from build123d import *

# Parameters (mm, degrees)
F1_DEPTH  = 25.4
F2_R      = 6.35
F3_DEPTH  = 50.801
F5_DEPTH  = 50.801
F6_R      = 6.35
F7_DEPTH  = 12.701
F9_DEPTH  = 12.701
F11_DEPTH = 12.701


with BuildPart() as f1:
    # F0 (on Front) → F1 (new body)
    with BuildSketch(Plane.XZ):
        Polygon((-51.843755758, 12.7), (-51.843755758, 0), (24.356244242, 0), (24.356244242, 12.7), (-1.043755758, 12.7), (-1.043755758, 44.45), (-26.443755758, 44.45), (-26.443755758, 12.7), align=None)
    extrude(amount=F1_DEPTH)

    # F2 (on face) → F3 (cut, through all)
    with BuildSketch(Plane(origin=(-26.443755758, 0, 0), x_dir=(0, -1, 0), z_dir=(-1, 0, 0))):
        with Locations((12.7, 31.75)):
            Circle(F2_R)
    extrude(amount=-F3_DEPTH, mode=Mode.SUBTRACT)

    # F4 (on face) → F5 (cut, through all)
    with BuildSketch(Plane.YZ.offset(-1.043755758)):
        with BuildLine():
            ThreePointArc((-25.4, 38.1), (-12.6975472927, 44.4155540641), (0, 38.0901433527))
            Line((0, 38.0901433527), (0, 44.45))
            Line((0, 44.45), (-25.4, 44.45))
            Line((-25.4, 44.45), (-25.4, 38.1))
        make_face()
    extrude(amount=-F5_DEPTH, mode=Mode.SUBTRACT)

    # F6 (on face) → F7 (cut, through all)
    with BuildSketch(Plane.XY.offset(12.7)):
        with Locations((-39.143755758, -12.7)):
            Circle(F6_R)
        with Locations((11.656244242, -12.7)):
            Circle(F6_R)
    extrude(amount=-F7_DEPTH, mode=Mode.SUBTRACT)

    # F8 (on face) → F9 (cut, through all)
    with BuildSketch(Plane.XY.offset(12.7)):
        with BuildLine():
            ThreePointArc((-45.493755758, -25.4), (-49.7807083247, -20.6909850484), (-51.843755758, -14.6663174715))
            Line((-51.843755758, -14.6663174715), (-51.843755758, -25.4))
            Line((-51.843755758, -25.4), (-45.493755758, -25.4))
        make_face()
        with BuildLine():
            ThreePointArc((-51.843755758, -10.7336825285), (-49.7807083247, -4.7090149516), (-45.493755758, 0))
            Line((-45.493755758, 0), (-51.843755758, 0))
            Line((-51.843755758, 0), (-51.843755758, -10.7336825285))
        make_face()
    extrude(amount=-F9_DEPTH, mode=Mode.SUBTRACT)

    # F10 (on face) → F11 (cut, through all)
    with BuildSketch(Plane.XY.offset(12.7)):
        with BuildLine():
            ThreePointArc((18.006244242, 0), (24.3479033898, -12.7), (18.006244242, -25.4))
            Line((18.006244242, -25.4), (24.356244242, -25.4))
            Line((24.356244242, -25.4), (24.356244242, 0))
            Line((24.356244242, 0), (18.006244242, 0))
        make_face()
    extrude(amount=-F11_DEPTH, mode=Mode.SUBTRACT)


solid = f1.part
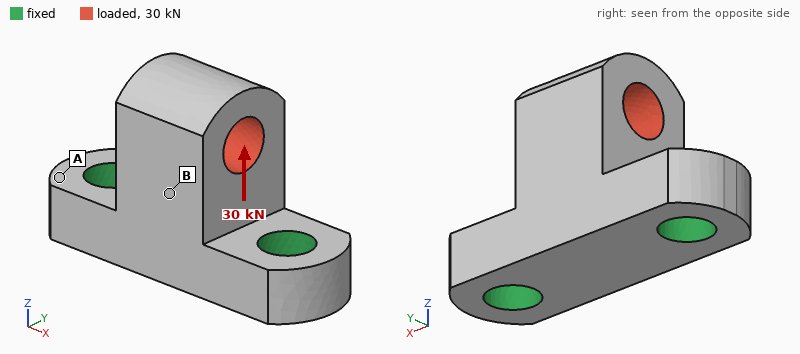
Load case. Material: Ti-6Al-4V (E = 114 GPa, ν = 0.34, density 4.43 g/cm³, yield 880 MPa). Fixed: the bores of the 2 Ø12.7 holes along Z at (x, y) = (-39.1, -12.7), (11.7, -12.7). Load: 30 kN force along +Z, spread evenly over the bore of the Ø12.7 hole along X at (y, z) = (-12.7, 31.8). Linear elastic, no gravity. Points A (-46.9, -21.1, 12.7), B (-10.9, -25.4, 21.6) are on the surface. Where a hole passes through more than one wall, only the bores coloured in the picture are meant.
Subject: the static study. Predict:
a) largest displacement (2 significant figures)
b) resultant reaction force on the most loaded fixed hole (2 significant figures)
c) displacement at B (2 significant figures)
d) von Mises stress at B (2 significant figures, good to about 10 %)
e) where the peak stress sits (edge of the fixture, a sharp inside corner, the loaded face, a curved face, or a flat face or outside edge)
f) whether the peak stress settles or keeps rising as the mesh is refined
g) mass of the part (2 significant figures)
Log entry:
42 µm
16 kN
27 µm
49 MPa
edge of the fixture
keeps rising
160 g
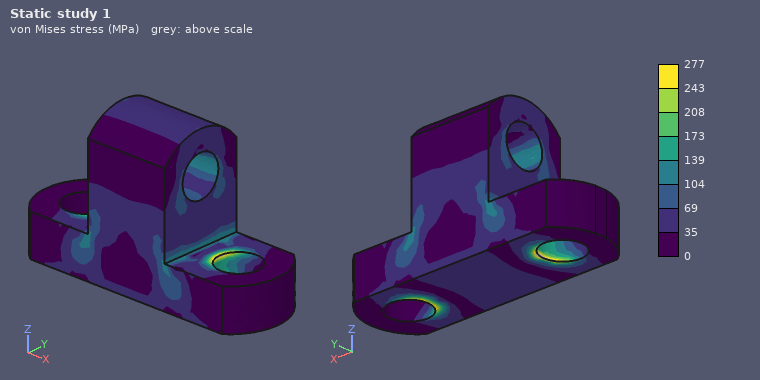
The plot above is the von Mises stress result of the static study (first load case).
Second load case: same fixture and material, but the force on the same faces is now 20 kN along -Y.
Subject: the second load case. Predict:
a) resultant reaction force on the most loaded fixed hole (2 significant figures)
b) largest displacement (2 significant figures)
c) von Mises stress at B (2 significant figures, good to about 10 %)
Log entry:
10 kN
0.27 mm
100 MPa
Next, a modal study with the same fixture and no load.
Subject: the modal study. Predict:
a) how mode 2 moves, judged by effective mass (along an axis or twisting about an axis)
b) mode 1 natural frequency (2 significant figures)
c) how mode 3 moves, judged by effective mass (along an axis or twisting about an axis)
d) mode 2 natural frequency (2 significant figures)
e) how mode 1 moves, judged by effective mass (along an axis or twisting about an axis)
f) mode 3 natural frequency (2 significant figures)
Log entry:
along X
6700 Hz
along Z
12 kHz
along Y
17 kHz
